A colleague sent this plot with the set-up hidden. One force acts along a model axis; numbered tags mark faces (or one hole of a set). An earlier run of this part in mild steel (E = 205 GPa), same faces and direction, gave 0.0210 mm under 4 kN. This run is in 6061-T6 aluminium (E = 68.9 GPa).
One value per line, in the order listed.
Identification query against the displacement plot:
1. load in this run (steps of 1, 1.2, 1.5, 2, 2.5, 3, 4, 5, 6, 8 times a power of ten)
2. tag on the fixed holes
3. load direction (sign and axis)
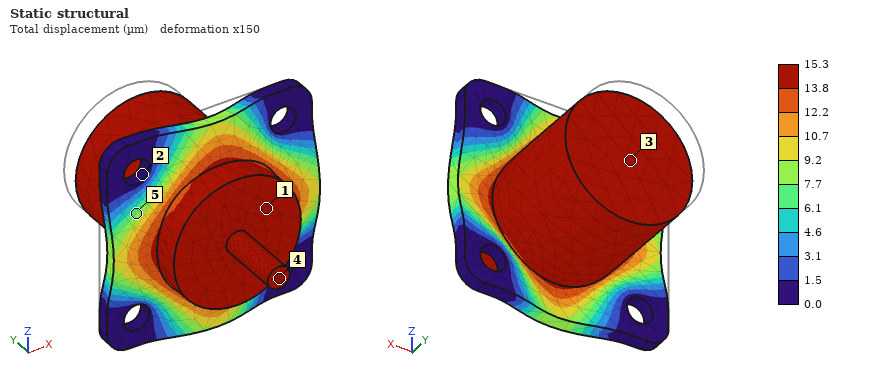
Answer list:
1 kN
2
-Y
